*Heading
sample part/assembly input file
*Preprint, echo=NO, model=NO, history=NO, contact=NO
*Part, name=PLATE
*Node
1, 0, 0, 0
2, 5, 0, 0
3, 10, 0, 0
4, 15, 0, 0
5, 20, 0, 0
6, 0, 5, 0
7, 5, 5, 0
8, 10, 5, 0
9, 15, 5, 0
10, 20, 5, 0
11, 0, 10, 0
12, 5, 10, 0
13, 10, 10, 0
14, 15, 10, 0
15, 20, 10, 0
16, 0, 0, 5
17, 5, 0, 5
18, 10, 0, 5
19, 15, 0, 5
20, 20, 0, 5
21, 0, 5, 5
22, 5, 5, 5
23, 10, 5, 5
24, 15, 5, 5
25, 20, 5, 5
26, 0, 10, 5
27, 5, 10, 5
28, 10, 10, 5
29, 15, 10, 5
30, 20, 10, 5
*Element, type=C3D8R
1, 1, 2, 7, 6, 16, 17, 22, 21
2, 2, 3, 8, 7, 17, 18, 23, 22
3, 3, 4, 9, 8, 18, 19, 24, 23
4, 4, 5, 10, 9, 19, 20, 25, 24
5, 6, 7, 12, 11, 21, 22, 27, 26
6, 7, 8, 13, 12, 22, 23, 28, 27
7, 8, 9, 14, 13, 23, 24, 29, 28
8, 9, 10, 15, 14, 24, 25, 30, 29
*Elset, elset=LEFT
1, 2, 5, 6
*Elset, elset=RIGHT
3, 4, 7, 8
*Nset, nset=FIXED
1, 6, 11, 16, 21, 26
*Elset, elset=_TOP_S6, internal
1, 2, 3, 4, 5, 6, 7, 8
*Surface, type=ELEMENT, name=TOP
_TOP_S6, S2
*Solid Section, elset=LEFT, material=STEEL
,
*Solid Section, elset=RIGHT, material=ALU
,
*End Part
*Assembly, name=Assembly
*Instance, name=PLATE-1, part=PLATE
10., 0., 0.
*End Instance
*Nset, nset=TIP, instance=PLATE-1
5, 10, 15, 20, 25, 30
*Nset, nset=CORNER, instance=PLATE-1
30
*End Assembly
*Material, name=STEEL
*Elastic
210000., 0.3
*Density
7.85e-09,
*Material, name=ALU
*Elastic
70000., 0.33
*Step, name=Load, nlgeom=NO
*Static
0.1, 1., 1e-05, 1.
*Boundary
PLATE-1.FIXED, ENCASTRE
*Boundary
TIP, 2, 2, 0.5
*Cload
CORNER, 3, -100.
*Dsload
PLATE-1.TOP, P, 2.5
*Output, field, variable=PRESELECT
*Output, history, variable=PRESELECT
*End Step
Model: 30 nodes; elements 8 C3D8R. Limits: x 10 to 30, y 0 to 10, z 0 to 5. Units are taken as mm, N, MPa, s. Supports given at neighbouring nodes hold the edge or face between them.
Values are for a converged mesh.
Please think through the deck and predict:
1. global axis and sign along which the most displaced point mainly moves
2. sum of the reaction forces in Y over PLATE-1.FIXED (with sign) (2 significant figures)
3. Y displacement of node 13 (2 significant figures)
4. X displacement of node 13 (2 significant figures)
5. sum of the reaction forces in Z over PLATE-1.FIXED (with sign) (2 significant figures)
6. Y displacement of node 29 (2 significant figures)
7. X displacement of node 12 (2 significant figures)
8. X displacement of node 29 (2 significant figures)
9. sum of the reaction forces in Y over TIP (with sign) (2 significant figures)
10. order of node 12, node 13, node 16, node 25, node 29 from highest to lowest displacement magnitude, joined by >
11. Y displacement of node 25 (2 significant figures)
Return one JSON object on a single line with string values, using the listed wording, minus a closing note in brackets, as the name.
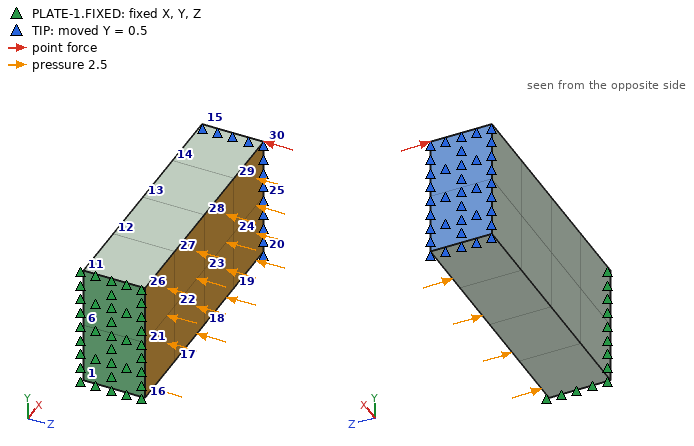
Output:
{"global axis and sign along which the most displaced point mainly moves": "+Y", "sum of the reaction forces in Y over PLATE-1.FIXED (with sign)": "-10000 N", "Y displacement of node 13": "0.13 mm", "X displacement of node 13": "-0.097 mm", "sum of the reaction forces in Z over PLATE-1.FIXED (with sign)": "600 N", "Y displacement of node 29": "0.29 mm", "X displacement of node 12": "-0.054 mm", "X displacement of node 29": "-0.15 mm", "sum of the reaction forces in Y over TIP (with sign)": "10000 N", "order of node 12, node 13, node 16, node 25, node 29 from highest to lowest displacement magnitude, joined by >": "node 25 > node 29 > node 13 > node 12 > node 16", "Y displacement of node 25": "0.50 mm"}
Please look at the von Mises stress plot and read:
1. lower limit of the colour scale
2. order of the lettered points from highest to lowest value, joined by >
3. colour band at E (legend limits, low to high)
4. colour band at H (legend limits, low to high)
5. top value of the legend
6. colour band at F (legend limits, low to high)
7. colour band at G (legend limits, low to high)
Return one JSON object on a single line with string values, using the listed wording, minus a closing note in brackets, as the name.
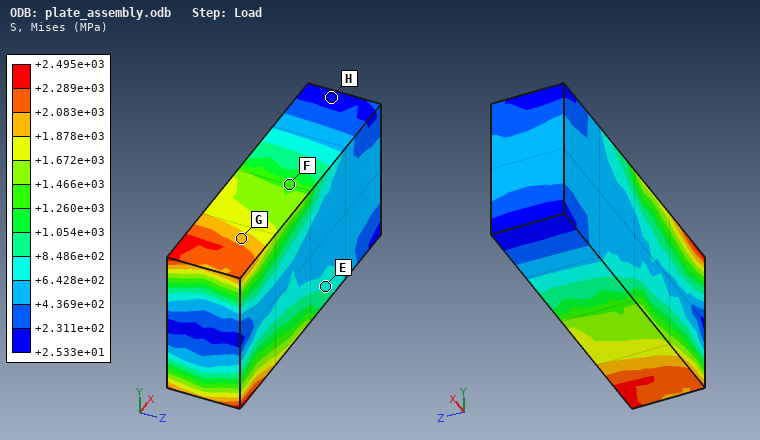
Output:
{"lower limit of the colour scale": "+2.533e+01 MPa", "order of the lettered points from highest to lowest value, joined by >": "G > F > E > H", "colour band at E": "+6.428e+02 to +8.486e+02 MPa", "colour band at H": "+2.533e+01 to +2.311e+02 MPa", "top value of the legend": "+2.495e+03 MPa", "colour band at F": "+1.260e+03 to +1.466e+03 MPa", "colour band at G": "+1.878e+03 to +2.083e+03 MPa"}
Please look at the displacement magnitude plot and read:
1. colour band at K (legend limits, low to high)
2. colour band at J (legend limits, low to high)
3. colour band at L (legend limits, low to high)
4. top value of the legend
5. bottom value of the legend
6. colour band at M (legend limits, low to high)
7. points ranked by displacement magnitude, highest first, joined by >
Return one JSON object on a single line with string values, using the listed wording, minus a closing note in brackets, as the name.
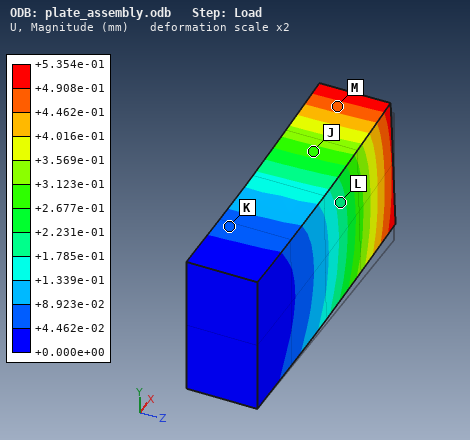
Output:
{"colour band at K": "+4.462e-02 to +8.923e-02 mm", "colour band at J": "+2.677e-01 to +3.123e-01 mm", "colour band at L": "+1.785e-01 to +2.231e-01 mm", "top value of the legend": "+5.354e-01 mm", "bottom value of the legend": "+0.000e+00 mm", "colour band at M": "+4.462e-01 to +4.908e-01 mm", "points ranked by displacement magnitude, highest first, joined by >": "M > J > L > K"}
